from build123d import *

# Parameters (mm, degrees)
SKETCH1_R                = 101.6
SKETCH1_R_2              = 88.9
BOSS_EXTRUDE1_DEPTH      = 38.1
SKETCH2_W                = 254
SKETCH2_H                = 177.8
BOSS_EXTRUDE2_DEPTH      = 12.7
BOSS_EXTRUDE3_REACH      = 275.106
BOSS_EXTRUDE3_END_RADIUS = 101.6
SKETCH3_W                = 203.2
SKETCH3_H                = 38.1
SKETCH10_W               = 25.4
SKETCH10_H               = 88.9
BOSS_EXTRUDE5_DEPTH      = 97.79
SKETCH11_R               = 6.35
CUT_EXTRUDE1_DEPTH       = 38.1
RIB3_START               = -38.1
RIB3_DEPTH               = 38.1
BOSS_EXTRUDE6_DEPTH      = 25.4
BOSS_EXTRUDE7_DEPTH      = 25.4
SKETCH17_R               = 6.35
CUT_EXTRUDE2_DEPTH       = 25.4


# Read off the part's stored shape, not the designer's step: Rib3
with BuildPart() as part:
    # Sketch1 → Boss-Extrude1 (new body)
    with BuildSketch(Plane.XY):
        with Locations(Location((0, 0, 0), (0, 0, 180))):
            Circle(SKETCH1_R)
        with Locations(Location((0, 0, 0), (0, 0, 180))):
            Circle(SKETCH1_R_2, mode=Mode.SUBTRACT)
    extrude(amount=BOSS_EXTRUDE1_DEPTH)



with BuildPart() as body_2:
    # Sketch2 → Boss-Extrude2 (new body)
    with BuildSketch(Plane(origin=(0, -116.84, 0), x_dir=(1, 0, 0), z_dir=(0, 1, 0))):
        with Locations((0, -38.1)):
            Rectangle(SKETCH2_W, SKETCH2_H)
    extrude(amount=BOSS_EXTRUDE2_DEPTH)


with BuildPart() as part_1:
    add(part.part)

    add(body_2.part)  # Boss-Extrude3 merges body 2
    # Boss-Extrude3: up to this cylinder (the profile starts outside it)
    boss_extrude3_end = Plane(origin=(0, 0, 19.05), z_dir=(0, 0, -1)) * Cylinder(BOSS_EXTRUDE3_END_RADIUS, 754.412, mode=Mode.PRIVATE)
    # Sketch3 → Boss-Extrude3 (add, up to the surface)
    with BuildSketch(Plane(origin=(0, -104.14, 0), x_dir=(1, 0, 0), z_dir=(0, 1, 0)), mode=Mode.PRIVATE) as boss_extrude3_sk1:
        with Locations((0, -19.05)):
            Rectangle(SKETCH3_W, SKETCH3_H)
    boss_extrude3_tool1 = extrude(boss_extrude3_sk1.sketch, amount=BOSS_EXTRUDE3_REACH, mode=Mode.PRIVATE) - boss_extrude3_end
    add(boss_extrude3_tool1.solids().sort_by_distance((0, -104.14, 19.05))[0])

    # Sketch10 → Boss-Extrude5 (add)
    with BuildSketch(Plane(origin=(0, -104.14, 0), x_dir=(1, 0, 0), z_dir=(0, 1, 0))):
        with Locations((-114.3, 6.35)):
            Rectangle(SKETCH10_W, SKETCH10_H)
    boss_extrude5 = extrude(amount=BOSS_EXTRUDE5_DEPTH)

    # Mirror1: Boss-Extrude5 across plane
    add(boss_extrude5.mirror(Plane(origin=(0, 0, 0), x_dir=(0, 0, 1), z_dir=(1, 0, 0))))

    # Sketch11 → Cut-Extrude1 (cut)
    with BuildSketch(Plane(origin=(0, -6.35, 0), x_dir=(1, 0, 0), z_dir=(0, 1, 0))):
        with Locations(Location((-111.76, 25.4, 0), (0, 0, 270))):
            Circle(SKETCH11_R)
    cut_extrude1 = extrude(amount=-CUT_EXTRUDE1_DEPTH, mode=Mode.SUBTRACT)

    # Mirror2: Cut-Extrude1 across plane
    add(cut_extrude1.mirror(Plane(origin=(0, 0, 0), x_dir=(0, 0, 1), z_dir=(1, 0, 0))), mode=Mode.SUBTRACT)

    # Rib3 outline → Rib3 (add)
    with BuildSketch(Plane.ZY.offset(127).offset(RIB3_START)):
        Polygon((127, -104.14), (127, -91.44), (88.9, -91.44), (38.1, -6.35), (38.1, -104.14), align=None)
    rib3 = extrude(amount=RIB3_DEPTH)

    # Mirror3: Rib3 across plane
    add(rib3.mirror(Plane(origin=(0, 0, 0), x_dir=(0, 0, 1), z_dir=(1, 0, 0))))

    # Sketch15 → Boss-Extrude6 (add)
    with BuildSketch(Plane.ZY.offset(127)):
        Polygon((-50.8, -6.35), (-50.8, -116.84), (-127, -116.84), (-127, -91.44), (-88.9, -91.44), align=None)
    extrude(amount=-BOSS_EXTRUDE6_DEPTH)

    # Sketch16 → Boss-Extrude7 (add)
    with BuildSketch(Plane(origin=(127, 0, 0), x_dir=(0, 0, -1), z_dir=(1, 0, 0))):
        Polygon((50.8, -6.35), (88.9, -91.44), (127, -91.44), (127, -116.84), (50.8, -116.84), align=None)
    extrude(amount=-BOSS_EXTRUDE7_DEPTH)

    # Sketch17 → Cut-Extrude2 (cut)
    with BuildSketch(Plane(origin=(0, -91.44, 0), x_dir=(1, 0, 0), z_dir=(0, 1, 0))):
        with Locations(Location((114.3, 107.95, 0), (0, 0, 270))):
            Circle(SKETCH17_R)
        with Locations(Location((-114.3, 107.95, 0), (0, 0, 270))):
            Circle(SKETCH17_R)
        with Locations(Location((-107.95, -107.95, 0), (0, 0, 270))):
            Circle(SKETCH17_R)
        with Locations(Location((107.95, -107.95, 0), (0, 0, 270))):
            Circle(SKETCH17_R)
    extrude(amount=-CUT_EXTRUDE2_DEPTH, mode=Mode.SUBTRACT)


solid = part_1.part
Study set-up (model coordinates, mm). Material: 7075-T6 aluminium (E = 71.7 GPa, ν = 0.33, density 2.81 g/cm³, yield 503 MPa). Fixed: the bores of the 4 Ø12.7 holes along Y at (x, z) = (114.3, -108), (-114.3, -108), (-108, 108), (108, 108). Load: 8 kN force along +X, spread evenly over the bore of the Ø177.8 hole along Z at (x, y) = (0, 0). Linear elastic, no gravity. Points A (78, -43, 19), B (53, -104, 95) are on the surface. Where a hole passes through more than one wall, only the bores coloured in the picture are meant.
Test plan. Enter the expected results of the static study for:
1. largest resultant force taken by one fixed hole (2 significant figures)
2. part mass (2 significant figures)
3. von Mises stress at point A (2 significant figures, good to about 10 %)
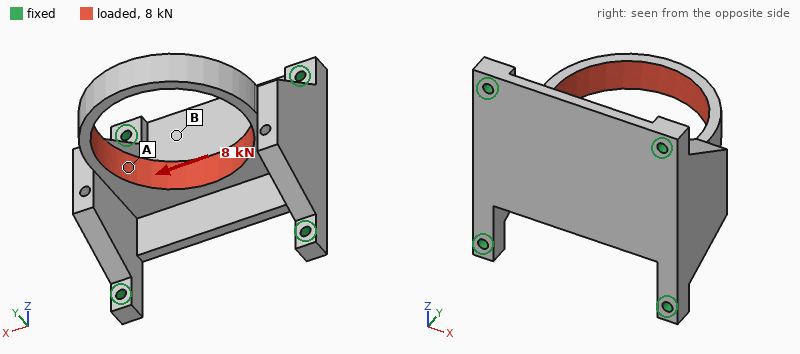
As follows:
5.1 kN
5.3 kg
9.1 MPa
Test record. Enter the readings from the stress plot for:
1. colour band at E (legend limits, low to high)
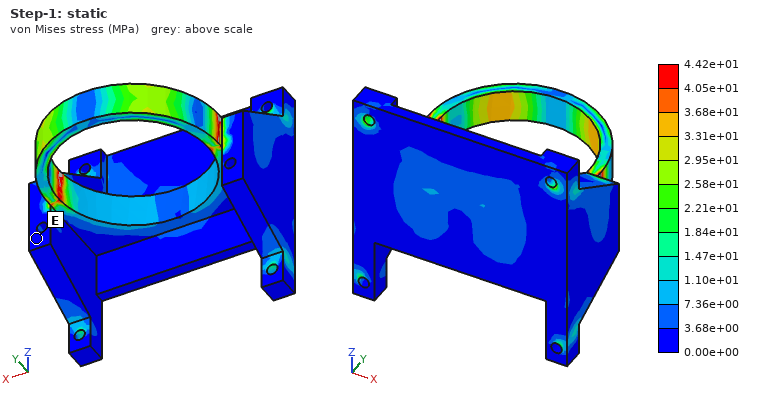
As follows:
0.00e+00 to 3.68e+00 MPa
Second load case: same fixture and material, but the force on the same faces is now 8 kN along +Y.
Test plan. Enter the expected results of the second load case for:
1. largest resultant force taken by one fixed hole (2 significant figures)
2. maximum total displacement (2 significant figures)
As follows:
2.7 kN
33 µm
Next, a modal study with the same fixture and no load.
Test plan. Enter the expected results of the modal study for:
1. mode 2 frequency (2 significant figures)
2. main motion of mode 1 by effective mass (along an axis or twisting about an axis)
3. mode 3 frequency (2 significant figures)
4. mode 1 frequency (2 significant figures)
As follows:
1100 Hz
along X
1200 Hz
1000 Hz
